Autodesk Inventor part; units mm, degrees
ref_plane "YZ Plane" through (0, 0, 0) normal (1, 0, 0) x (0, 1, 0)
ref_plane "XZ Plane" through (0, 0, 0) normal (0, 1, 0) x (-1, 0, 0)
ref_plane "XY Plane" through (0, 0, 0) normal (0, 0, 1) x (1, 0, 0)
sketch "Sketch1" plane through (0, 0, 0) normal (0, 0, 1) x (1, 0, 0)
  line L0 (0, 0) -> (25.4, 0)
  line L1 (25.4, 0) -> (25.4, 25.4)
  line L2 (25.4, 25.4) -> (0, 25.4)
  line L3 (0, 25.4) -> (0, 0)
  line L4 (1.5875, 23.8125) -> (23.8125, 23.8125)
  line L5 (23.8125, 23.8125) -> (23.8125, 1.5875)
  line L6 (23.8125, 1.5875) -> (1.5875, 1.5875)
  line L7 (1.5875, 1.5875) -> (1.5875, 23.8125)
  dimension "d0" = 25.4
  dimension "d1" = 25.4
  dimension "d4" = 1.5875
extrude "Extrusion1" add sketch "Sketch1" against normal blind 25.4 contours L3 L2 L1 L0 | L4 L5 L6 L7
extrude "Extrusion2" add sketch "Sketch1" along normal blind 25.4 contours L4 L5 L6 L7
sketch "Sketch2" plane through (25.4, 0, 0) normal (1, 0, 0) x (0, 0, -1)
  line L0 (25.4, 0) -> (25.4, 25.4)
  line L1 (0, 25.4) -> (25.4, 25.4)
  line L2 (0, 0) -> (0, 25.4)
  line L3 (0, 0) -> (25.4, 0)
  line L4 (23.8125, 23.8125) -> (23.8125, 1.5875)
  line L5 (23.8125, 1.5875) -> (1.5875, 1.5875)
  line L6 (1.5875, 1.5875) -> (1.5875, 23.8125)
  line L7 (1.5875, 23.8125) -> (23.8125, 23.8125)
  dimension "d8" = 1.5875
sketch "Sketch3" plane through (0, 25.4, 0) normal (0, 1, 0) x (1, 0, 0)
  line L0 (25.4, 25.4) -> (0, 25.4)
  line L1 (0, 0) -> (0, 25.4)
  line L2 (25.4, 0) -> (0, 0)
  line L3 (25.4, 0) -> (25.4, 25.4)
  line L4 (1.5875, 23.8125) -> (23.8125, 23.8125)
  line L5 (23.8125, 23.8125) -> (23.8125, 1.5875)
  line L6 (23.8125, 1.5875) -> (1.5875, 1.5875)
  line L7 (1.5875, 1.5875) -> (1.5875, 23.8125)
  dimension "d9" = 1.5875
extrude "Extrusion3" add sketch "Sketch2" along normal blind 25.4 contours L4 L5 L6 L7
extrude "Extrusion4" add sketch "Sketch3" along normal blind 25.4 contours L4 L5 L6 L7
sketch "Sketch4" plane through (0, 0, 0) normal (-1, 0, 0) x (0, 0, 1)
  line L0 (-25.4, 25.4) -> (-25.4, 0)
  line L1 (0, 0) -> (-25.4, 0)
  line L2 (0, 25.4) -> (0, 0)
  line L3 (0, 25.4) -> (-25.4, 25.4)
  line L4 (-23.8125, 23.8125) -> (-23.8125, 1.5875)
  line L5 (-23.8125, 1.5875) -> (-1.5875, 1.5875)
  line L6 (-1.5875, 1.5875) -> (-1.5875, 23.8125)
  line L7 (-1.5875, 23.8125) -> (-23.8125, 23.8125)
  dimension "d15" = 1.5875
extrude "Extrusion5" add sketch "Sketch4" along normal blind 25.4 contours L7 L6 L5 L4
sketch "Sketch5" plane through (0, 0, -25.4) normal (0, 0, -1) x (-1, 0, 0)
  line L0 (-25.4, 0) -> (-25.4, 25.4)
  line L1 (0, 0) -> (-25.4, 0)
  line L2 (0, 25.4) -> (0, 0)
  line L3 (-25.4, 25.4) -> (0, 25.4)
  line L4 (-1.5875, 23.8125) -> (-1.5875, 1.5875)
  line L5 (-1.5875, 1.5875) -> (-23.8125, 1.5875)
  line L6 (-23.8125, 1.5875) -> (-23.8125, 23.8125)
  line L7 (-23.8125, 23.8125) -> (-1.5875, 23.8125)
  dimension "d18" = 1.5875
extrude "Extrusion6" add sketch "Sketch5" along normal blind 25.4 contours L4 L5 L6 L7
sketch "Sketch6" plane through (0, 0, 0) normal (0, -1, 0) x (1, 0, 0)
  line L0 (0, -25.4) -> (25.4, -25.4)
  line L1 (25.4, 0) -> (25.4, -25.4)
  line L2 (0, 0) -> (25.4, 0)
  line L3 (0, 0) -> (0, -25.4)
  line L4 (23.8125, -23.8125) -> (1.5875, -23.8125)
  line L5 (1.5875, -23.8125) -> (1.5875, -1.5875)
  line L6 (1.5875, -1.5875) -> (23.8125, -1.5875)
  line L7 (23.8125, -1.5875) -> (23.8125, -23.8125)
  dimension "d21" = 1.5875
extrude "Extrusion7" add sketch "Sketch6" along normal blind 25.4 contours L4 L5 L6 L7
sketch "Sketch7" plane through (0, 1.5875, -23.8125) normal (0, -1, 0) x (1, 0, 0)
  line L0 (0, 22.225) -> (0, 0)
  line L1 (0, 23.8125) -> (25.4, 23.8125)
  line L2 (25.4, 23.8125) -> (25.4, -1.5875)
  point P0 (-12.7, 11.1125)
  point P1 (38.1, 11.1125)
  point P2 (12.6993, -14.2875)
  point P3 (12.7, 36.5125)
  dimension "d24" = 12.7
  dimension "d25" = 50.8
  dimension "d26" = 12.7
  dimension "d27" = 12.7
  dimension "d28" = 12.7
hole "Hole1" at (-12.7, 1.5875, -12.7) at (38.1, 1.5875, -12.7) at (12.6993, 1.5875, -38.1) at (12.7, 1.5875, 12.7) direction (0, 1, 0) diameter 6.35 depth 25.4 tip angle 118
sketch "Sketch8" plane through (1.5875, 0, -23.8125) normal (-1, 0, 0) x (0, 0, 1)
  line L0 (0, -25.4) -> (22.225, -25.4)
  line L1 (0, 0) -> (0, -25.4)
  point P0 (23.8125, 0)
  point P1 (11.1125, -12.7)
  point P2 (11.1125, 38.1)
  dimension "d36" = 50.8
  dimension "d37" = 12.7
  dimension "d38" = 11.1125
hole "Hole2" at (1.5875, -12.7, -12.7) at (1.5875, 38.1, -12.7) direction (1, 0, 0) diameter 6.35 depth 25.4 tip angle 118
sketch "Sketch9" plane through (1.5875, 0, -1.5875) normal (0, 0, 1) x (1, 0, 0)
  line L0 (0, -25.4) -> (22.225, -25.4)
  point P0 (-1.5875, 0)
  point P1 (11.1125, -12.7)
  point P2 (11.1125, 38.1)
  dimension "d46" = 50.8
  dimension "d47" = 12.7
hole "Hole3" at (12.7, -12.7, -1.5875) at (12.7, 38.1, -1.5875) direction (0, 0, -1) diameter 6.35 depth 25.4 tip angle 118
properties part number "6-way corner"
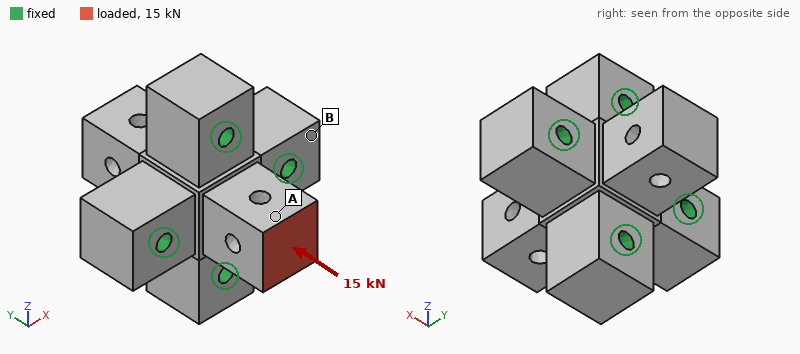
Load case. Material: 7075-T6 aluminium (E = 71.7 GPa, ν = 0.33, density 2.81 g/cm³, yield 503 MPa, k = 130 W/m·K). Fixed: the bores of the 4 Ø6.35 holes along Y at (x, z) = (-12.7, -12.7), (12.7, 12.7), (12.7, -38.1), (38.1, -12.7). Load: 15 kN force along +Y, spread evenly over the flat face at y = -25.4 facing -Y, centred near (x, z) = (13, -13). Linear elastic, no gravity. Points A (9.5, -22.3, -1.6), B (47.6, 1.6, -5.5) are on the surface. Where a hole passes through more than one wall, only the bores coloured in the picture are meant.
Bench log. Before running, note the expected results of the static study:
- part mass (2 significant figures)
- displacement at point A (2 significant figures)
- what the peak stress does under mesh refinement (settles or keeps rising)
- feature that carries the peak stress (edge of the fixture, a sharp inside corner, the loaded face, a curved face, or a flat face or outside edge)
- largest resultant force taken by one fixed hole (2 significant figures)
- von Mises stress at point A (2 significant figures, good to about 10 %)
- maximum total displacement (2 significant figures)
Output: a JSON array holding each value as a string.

["240 g", "21 µm", "keeps rising", "a sharp inside corner", "3.9 kN", "33 MPa", "24 µm"]
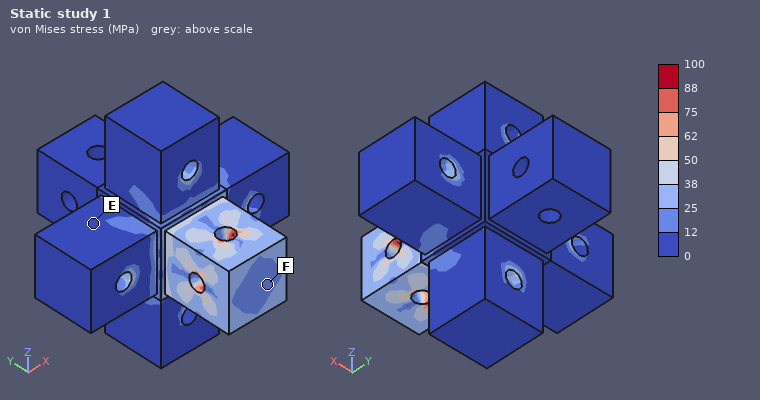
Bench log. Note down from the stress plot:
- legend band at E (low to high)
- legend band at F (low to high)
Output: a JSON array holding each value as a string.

["0 to 12 MPa", "12 to 25 MPa"]
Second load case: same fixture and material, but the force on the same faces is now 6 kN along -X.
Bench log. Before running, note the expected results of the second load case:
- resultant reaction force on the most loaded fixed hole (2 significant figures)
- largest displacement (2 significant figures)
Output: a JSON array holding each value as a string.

["5.2 kN", "78 µm"]
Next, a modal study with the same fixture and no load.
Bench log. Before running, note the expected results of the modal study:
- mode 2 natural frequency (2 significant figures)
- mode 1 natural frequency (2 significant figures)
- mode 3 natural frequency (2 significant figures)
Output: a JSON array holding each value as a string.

["13 kHz", "13 kHz", "14 kHz"]
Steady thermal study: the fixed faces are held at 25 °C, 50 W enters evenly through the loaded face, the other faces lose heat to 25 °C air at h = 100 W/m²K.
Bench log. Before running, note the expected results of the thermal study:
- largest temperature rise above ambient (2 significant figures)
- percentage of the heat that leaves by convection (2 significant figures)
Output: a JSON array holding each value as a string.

["30 K", "13 %"]
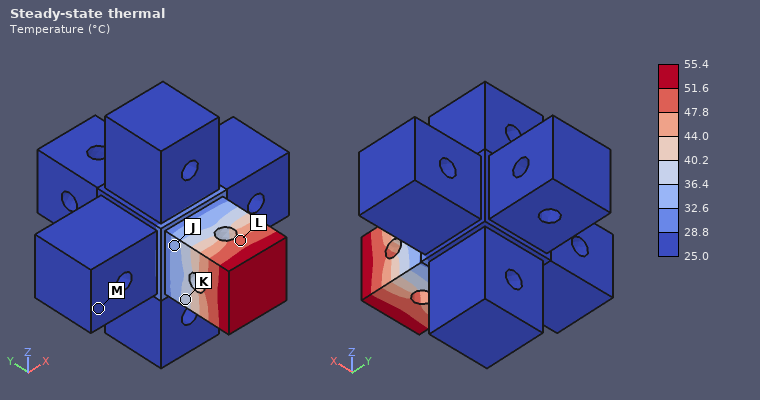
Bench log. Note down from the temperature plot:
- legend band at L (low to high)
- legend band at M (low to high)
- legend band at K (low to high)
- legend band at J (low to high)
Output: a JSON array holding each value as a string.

["47.8 to 51.6 °C", "25.0 to 28.8 °C", "36.4 to 40.2 °C", "32.6 to 36.4 °C"]
